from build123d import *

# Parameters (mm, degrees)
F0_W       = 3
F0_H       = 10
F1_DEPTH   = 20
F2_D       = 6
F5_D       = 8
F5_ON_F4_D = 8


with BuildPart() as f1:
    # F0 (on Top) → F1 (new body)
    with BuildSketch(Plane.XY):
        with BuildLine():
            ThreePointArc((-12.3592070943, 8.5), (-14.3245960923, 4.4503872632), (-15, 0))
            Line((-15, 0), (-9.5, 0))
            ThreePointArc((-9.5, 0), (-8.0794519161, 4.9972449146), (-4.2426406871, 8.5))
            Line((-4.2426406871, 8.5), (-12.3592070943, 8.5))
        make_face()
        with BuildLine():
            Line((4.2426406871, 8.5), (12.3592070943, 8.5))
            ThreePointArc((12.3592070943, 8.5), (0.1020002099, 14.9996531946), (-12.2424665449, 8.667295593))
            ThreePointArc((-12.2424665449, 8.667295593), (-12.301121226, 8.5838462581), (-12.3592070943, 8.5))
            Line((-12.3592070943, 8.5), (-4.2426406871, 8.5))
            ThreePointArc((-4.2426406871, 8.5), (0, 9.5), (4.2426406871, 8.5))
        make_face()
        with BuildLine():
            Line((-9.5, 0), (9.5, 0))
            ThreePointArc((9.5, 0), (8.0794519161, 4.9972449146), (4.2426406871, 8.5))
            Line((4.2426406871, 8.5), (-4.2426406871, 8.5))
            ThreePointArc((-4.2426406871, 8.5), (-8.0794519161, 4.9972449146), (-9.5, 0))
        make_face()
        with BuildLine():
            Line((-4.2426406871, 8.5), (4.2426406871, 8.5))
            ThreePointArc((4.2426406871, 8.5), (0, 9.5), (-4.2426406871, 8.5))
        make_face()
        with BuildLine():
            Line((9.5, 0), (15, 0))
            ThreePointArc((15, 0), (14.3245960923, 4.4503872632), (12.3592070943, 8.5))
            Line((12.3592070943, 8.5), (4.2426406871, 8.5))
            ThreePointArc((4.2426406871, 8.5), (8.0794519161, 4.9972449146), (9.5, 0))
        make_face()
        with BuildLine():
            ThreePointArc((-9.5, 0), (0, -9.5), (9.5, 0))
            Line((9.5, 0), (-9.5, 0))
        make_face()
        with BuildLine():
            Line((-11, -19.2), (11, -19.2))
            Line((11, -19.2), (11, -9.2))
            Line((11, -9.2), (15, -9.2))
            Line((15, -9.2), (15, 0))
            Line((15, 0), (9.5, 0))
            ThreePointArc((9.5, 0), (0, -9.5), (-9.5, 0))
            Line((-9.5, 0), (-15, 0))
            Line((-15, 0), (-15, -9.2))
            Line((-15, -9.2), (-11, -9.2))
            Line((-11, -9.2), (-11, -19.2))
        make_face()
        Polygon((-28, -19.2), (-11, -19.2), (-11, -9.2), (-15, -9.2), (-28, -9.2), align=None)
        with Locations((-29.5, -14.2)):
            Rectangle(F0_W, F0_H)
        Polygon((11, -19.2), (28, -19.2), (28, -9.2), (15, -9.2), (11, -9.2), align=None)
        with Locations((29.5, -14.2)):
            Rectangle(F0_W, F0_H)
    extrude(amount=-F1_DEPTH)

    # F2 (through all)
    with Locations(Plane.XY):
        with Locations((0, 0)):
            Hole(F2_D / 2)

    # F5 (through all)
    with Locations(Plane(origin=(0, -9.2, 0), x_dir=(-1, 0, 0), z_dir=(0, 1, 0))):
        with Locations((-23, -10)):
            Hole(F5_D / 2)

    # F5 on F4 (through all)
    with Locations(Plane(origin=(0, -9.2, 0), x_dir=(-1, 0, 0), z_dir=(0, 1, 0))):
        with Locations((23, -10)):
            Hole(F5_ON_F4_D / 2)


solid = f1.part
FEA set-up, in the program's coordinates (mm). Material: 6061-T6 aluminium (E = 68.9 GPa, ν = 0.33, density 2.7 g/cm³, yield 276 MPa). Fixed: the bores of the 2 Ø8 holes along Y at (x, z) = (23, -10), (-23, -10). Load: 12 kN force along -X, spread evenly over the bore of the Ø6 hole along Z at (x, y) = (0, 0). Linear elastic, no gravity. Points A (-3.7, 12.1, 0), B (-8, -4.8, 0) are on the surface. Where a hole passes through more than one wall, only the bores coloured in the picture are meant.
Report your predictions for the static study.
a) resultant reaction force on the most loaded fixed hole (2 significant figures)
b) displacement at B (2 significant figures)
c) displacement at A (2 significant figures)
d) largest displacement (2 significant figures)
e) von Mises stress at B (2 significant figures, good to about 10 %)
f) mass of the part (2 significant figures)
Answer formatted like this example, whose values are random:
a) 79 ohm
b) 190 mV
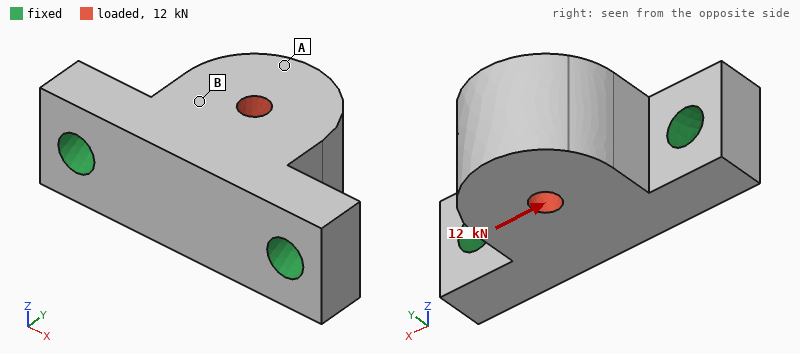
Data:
a) 7.5 kN
b) 15 µm
c) 33 µm
d) 34 µm
e) 44 MPa
f) 63 g
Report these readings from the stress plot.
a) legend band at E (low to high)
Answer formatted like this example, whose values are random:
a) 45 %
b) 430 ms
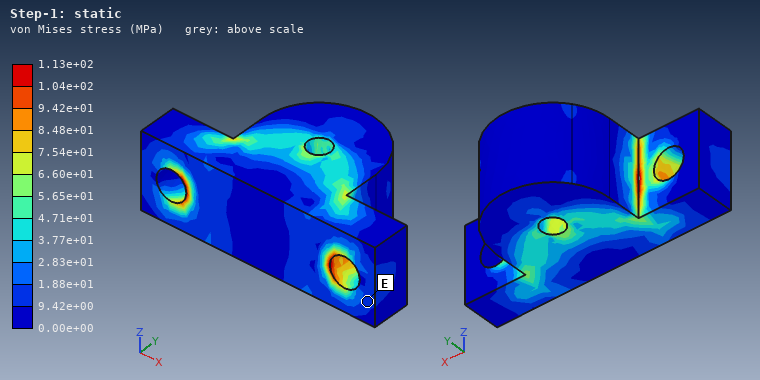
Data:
a) 9.42e+00 to 1.88e+01 MPa
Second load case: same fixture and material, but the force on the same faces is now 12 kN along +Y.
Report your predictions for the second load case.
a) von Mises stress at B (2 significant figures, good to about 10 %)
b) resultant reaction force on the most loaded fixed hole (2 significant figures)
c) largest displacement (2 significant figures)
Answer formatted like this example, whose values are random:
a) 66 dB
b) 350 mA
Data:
a) 29 MPa
b) 6.5 kN
c) 25 µm
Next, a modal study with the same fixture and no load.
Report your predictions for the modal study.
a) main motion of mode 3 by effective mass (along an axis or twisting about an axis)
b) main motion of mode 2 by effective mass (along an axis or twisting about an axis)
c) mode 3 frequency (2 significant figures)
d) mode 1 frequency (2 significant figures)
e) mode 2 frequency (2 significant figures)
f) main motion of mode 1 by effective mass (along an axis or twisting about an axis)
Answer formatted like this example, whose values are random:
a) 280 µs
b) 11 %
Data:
a) along Y
b) along X
c) 18 kHz
d) 7500 Hz
e) 17 kHz
f) along Z
